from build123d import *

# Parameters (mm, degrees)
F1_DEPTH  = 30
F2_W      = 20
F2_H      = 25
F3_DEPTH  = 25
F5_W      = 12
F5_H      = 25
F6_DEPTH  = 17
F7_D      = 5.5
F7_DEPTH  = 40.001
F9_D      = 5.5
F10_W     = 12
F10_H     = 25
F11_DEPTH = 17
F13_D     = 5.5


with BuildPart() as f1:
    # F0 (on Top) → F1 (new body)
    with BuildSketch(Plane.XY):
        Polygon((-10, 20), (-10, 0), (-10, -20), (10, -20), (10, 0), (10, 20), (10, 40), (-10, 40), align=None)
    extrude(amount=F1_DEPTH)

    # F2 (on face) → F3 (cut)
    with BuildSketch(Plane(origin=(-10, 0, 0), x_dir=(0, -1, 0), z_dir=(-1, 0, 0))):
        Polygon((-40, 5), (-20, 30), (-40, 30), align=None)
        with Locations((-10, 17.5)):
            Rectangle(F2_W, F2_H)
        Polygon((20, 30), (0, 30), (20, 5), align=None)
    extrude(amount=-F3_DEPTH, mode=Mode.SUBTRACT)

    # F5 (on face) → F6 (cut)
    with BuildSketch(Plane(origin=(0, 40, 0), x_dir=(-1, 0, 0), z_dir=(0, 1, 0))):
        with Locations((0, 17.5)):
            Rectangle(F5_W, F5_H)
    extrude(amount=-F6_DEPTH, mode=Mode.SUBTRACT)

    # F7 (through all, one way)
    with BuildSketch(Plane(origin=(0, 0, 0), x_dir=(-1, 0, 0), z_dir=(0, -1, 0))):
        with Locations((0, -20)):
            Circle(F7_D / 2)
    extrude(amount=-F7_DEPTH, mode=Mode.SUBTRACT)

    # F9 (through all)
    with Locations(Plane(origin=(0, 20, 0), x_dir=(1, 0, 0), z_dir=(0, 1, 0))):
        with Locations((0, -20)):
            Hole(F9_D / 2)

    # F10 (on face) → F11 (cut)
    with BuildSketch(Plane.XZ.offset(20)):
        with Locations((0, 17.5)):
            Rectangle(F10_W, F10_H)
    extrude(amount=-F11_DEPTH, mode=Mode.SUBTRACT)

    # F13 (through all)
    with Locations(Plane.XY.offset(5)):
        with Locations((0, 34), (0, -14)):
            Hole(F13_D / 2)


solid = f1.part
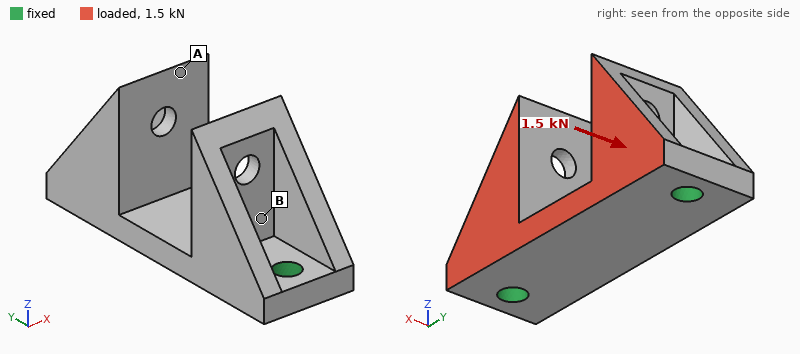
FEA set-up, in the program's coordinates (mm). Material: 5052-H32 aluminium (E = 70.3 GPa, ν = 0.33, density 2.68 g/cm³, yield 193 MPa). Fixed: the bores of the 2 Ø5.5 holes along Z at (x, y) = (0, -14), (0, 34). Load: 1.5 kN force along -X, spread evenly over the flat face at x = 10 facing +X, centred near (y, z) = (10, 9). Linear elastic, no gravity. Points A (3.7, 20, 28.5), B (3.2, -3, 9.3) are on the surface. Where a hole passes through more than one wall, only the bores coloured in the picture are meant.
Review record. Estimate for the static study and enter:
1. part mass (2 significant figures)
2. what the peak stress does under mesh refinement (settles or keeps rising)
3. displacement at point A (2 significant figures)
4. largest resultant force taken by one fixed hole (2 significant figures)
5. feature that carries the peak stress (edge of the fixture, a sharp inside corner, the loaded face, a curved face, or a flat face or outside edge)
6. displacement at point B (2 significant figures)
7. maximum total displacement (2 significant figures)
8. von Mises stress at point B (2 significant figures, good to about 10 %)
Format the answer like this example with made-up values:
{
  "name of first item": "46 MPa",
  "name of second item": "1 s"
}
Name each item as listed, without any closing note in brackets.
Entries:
{
  "part mass": "30 g",
  "what the peak stress does under mesh refinement": "keeps rising",
  "displacement at point A": "40 µm",
  "largest resultant force taken by one fixed hole": "750 N",
  "feature that carries the peak stress": "edge of the fixture",
  "displacement at point B": "14 µm",
  "maximum total displacement": "46 µm",
  "von Mises stress at point B": "16 MPa"
}
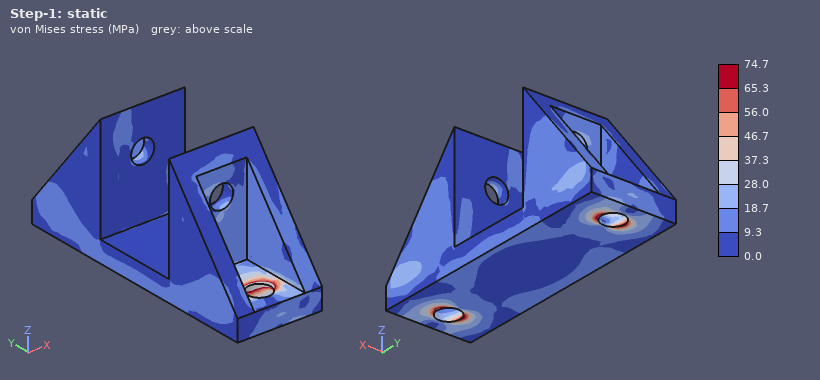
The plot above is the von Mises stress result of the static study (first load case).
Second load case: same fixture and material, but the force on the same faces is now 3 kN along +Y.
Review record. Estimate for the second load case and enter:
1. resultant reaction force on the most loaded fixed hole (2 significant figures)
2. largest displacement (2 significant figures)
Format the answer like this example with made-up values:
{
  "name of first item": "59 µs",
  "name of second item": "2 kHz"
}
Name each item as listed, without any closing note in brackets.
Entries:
{
  "resultant reaction force on the most loaded fixed hole": "1.6 kN",
  "largest displacement": "51 µm"
}
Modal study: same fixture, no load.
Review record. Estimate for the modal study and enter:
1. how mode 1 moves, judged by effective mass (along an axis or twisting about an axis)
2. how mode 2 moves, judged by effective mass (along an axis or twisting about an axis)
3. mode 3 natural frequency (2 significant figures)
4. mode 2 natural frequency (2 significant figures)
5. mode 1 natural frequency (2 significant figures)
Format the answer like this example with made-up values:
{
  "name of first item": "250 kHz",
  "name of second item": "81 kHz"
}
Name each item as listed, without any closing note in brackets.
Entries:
{
  "how mode 1 moves, judged by effective mass": "along X",
  "how mode 2 moves, judged by effective mass": "along Z",
  "mode 3 natural frequency": "9000 Hz",
  "mode 2 natural frequency": "7400 Hz",
  "mode 1 natural frequency": "6900 Hz"
}
